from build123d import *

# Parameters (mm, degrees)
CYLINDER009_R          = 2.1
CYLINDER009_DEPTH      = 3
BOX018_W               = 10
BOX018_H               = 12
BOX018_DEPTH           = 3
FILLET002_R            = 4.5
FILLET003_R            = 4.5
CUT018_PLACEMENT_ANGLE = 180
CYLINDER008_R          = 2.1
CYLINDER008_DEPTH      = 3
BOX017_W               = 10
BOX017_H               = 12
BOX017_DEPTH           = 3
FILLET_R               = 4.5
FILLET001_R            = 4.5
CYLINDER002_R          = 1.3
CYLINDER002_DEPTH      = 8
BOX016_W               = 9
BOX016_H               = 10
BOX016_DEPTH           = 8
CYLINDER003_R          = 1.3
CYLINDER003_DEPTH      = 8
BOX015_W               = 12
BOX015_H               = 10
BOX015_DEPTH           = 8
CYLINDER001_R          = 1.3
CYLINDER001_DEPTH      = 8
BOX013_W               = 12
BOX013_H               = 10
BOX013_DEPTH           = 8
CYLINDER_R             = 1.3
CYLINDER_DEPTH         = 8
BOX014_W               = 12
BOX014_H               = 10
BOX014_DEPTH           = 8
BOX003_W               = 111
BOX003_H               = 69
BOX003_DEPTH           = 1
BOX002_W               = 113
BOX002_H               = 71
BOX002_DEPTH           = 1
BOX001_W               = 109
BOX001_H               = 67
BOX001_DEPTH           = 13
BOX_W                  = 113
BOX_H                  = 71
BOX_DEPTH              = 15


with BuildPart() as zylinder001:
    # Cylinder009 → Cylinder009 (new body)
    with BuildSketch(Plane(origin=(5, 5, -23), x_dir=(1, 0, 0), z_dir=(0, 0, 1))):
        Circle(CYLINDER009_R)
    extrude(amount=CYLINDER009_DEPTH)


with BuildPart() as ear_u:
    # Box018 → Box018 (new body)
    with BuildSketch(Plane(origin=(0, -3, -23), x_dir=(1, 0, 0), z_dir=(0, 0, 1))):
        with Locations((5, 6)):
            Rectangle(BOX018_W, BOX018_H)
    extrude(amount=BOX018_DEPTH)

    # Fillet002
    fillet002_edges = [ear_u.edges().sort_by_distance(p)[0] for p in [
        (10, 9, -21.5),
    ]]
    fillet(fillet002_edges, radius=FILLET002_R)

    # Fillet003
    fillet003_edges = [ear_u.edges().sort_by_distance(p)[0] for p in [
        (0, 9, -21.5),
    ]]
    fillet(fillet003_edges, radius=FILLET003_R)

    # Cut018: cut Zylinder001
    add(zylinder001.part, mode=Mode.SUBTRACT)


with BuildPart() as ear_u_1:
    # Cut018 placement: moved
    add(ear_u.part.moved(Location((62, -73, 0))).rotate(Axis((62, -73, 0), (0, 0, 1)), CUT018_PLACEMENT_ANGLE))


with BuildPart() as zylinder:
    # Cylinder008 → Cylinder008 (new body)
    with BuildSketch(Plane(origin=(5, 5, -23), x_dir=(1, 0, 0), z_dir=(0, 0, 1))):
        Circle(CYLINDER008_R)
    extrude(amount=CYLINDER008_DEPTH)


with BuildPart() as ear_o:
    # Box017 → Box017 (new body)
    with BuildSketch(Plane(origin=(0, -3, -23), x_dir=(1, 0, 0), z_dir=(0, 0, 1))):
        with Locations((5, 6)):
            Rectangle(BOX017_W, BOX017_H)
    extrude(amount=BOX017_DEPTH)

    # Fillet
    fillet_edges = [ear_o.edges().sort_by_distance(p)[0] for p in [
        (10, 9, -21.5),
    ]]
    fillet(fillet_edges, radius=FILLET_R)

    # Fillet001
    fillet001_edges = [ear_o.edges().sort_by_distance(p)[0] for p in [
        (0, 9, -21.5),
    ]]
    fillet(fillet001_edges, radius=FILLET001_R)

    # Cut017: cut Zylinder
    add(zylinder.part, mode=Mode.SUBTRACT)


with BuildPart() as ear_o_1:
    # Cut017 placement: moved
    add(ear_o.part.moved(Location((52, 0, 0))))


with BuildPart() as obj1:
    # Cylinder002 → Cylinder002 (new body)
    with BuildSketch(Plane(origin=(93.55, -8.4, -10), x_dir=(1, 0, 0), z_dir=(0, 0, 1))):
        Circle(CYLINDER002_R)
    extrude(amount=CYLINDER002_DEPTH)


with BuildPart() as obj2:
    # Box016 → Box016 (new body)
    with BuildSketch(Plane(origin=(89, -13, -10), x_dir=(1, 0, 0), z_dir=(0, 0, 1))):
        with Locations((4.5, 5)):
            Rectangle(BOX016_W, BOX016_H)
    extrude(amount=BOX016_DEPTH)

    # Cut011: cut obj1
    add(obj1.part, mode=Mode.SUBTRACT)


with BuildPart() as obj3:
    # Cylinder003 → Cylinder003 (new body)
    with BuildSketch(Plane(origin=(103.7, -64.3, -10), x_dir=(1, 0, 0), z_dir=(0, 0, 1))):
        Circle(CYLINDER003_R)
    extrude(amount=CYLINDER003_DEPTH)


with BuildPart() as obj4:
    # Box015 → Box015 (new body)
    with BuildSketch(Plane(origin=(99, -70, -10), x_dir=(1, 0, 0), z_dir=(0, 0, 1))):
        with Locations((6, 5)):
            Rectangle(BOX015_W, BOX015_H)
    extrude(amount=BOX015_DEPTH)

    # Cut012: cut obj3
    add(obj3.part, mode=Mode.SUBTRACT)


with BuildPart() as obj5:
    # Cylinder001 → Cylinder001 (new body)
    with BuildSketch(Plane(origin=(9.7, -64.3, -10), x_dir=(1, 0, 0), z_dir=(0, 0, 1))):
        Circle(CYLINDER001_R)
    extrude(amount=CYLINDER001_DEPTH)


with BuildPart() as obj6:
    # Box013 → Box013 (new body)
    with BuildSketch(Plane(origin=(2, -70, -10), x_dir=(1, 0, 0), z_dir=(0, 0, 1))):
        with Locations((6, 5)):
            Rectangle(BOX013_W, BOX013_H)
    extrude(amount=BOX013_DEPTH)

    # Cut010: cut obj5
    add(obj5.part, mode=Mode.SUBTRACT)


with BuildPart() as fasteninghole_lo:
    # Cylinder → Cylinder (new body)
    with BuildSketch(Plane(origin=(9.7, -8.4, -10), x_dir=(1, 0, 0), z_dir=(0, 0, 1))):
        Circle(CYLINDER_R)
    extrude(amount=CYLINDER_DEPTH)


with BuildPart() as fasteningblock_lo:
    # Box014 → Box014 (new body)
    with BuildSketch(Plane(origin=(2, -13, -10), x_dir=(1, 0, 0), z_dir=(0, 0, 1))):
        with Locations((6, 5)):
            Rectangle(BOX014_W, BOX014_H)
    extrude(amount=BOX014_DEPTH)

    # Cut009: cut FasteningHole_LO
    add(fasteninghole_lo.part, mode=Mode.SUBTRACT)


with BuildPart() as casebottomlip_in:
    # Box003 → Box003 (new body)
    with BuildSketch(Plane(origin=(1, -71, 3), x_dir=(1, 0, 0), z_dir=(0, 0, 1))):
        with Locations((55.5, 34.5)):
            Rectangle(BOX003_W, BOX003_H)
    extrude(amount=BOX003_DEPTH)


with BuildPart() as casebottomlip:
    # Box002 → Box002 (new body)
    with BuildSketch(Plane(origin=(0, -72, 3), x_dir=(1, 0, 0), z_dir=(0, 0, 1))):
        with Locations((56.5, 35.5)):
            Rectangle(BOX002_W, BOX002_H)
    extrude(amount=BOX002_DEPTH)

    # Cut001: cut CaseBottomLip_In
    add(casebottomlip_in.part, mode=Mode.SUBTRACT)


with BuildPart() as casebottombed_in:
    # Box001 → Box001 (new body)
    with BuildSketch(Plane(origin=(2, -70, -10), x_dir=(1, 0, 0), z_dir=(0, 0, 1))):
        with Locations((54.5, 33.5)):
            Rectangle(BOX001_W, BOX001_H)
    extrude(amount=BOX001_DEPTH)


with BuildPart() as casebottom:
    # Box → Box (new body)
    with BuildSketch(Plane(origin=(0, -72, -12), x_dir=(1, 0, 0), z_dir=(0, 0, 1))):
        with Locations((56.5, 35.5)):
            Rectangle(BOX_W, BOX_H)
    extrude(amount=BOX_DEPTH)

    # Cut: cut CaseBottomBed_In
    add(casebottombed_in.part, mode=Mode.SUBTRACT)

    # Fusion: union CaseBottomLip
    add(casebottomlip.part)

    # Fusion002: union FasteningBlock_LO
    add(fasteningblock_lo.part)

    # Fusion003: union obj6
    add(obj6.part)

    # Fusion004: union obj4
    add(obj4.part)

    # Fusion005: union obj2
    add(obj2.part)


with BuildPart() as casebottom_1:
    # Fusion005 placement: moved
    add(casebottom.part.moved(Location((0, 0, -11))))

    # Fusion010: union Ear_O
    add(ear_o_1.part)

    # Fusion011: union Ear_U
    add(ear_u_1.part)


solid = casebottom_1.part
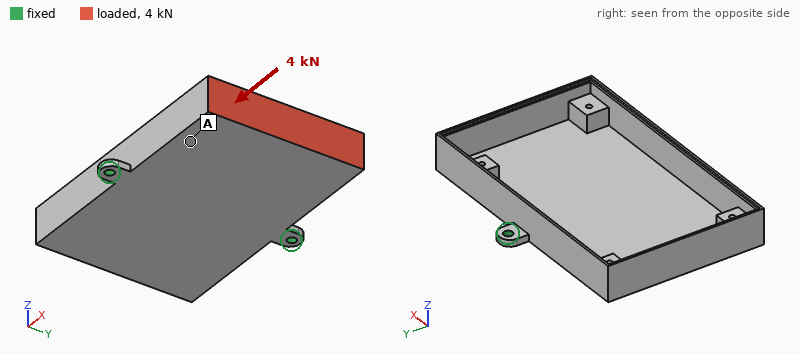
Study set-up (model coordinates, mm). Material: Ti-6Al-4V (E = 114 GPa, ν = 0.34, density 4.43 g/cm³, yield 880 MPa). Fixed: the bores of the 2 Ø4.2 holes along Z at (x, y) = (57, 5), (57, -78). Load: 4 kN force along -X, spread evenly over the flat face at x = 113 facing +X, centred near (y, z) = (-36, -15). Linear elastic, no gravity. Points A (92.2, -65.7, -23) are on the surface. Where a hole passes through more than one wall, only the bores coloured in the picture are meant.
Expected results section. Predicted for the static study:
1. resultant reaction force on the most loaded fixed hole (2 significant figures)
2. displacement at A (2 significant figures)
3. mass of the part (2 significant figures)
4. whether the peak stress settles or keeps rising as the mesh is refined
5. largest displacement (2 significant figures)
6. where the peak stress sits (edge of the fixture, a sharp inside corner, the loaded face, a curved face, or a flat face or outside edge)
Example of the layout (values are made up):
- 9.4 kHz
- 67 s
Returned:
- 2.0 kN
- 0.64 mm
- 130 g
- keeps rising
- 1.3 mm
- edge of the fixture
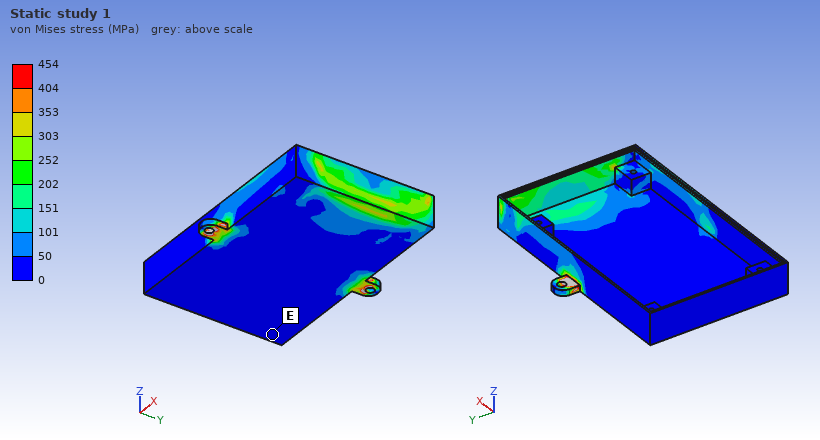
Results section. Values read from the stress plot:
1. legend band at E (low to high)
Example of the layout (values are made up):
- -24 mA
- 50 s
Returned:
- 0 to 50 MPa
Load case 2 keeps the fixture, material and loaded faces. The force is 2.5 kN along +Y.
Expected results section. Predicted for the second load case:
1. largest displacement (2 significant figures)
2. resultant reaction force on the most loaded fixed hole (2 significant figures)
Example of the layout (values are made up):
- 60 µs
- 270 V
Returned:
- 0.66 mm
- 2.2 kN
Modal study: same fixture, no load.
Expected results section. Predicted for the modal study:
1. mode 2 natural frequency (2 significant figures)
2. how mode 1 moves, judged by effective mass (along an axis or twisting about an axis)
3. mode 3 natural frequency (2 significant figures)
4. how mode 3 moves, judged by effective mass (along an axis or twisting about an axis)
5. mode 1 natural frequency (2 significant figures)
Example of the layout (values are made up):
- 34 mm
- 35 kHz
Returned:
- 950 Hz
- twisting about Y
- 1600 Hz
- along Z
- 440 Hz
